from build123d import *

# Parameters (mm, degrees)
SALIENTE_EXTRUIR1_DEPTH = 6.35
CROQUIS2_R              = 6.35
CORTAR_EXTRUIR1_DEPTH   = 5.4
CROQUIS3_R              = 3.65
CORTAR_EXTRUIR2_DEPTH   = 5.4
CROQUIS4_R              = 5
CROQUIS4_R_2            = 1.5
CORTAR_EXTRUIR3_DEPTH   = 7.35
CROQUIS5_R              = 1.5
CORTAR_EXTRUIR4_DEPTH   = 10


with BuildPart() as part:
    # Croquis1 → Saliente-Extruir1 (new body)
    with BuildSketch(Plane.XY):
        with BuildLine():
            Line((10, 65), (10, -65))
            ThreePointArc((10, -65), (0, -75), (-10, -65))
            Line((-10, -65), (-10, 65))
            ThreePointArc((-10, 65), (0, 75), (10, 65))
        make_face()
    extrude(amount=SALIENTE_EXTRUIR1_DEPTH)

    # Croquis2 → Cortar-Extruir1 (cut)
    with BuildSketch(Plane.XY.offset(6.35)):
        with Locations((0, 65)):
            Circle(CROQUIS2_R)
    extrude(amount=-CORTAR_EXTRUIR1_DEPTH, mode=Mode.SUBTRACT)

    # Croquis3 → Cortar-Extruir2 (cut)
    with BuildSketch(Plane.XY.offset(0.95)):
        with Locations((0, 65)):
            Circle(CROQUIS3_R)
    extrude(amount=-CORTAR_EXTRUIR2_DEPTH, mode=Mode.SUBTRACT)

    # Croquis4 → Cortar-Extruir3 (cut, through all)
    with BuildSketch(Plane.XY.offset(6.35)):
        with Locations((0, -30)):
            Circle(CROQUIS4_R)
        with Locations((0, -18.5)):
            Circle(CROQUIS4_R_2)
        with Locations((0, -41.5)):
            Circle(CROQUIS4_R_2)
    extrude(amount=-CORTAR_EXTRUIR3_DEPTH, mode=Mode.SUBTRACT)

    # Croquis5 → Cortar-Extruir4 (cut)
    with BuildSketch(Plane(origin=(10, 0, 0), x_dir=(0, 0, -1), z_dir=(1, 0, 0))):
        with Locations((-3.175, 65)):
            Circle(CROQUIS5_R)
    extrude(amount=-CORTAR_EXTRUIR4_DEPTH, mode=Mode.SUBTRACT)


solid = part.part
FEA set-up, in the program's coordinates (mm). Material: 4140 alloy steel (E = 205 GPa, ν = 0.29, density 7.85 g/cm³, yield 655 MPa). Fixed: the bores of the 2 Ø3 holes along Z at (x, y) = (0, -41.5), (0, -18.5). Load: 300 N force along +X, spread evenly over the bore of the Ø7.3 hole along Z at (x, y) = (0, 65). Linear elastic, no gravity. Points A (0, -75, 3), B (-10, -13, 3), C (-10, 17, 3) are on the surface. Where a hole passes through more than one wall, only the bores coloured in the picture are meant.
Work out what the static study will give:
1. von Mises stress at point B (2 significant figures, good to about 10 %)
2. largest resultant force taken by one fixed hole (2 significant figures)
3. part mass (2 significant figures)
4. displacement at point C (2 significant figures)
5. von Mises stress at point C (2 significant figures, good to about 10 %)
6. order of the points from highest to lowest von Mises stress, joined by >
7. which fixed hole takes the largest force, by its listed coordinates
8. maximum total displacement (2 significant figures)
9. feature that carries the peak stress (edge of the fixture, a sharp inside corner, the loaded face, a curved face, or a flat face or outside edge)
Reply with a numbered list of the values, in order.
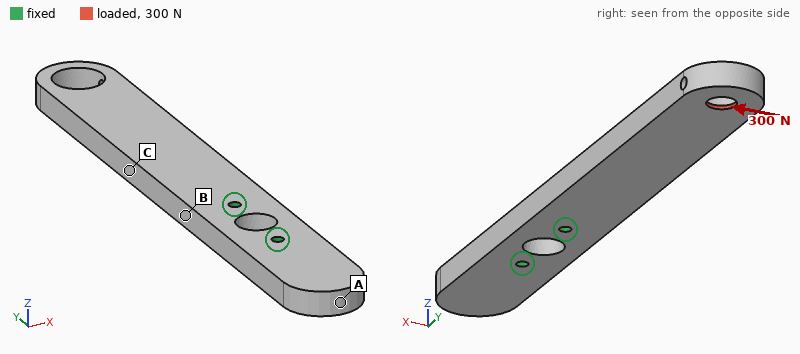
1. 57 MPa
2. 1.0 kN
3. 130 g
4. 0.035 mm
5. 34 MPa
6. B > C > A
7. (0, -18.5)
8. 0.12 mm
9. edge of the fixture
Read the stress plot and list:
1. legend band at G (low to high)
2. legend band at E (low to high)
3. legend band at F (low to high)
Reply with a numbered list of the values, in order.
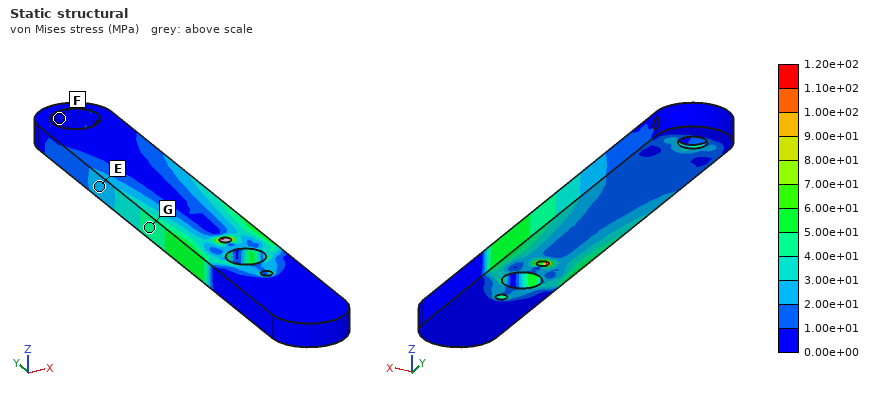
1. 4.00e+01 to 5.00e+01 MPa
2. 2.00e+01 to 3.00e+01 MPa
3. 0.00e+00 to 1.00e+01 MPa
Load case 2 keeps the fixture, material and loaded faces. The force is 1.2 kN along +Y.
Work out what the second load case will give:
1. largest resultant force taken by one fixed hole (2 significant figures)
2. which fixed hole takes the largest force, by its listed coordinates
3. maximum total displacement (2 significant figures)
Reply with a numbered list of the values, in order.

1. 1.0 kN
2. (0, -18.5)
3. 0.17 mm
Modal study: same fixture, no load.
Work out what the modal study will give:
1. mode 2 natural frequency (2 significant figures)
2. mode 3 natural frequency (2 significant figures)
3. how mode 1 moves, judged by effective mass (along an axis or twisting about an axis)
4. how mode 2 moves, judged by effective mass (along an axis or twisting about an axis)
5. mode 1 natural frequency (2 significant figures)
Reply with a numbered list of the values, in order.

1. 1700 Hz
2. 3900 Hz
3. along Z
4. along X
5. 680 Hz
